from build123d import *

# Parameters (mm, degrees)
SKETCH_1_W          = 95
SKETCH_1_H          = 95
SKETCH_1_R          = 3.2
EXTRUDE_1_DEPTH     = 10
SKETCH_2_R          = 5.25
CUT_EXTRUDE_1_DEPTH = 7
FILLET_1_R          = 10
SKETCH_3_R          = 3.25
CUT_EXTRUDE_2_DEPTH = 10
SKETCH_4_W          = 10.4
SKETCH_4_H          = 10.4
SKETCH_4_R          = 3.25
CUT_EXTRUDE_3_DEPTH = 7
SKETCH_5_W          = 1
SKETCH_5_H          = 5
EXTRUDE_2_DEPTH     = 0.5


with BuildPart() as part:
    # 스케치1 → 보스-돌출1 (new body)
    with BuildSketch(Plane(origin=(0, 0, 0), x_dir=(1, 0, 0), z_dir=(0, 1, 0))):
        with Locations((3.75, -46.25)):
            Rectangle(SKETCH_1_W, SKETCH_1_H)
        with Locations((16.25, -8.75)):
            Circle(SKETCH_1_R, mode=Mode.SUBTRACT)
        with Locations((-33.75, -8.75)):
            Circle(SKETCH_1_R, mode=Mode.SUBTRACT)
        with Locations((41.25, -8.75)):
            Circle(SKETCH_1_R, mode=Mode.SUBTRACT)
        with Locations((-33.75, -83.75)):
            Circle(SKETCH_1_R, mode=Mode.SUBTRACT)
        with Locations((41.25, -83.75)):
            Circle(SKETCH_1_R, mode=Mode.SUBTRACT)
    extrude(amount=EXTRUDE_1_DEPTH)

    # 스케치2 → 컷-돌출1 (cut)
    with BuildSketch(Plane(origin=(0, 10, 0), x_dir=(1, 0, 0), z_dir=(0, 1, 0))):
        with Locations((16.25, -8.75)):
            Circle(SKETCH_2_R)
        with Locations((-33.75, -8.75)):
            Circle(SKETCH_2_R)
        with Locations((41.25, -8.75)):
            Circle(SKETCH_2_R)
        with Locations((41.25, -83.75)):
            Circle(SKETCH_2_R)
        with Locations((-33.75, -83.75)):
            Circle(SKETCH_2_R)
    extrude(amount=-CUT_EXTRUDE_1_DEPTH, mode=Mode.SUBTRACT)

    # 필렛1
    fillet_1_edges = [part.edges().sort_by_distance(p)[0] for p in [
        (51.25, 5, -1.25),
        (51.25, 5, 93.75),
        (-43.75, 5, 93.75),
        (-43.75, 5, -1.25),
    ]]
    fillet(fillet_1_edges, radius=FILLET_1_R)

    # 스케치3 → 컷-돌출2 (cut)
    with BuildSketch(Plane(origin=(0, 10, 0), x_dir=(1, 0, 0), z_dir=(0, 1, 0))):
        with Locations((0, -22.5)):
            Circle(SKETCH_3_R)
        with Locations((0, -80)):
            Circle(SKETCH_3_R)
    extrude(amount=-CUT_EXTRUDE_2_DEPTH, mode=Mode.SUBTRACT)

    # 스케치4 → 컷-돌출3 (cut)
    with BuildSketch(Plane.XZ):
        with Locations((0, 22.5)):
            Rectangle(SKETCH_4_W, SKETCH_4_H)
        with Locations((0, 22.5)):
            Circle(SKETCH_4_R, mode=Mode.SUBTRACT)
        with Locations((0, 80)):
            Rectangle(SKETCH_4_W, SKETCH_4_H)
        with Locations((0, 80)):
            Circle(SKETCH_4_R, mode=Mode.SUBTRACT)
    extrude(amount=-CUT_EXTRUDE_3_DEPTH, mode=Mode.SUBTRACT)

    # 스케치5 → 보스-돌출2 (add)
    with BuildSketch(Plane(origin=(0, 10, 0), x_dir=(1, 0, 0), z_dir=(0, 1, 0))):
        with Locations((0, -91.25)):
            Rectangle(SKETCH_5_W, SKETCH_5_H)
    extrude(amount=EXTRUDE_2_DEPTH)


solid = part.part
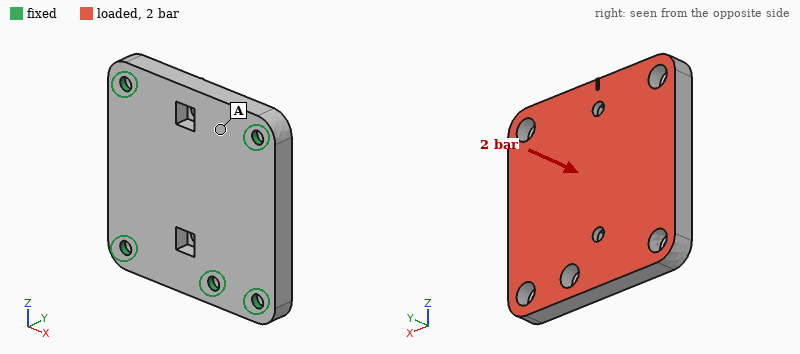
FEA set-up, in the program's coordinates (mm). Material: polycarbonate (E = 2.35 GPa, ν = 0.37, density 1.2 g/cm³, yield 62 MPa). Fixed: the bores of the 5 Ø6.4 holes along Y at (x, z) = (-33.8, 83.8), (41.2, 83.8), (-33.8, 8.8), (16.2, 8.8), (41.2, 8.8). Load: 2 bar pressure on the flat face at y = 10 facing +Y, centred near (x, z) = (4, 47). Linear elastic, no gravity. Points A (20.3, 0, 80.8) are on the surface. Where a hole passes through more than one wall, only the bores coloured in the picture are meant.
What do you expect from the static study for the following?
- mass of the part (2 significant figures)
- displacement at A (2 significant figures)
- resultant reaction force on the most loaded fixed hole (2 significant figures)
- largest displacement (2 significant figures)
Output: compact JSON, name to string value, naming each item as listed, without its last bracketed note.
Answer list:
{"mass of the part": "100 g", "displacement at A": "0.18 mm", "resultant reaction force on the most loaded fixed hole": "620 N", "largest displacement": "0.29 mm"}
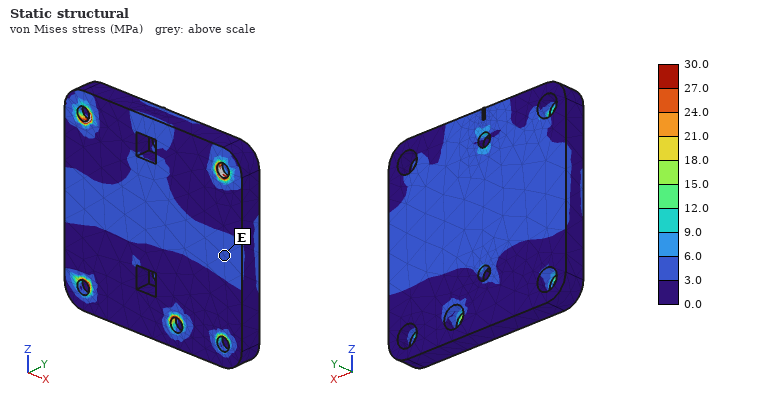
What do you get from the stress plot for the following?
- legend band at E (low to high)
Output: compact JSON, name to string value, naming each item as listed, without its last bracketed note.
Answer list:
{"legend band at E": "3.0 to 6.0 MPa"}
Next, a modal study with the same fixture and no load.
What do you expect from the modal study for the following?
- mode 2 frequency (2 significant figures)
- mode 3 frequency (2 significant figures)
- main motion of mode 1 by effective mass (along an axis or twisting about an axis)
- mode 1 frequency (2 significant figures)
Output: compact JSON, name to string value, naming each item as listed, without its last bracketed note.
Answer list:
{"mode 2 frequency": "2000 Hz", "mode 3 frequency": "2000 Hz", "main motion of mode 1 by effective mass": "along Y", "mode 1 frequency": "1400 Hz"}
